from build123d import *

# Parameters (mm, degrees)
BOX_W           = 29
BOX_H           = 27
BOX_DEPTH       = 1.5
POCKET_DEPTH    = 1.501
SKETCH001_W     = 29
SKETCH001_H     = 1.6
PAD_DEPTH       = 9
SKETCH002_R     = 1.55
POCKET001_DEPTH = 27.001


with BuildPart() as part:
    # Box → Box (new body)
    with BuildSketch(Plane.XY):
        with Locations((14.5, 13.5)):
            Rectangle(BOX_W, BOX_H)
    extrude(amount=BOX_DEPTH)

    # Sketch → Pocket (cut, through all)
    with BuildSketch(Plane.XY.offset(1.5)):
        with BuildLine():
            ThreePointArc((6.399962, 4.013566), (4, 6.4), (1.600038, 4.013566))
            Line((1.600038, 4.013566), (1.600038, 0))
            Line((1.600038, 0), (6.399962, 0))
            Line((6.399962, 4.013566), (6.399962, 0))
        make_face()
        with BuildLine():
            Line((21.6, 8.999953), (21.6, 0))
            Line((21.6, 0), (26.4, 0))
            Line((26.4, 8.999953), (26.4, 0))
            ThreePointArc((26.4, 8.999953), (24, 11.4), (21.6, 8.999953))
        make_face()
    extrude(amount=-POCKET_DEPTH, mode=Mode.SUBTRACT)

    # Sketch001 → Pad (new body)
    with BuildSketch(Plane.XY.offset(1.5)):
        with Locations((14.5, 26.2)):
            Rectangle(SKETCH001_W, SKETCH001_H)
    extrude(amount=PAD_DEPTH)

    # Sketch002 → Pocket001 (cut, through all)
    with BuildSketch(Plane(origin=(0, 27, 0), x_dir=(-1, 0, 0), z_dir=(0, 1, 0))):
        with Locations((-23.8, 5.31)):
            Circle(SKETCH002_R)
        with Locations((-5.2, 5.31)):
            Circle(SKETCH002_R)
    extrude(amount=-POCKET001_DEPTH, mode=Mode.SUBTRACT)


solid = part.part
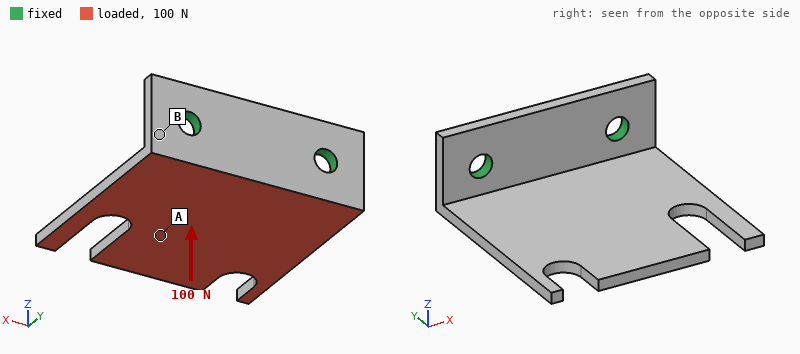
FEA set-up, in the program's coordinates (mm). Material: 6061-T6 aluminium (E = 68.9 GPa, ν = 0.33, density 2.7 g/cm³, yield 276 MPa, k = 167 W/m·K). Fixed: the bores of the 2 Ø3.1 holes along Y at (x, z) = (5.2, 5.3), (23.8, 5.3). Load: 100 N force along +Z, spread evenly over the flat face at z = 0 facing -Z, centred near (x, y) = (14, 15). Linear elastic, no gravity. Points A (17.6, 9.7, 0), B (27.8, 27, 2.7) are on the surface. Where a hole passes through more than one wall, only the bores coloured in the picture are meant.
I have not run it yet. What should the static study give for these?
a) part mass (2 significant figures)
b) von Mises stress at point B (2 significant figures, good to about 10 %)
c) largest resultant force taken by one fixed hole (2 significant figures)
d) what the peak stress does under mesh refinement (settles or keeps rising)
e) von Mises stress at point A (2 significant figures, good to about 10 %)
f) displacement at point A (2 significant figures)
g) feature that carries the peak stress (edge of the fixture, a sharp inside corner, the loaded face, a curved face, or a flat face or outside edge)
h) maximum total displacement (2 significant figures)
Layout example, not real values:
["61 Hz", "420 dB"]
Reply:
["3.9 g", "76 MPa", "52 N", "keeps rising", "17 MPa", "0.27 mm", "edge of the fixture", "0.48 mm"]
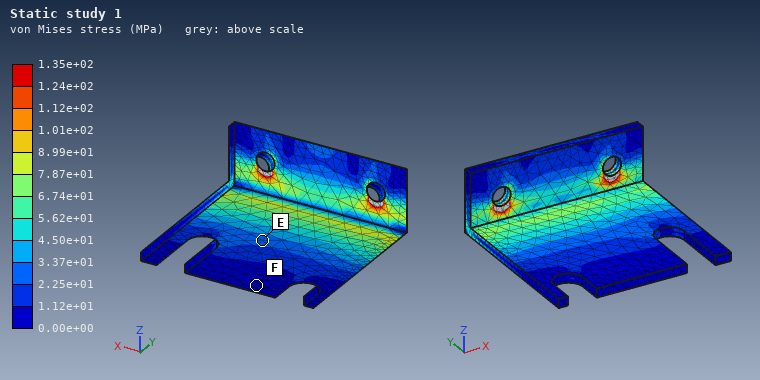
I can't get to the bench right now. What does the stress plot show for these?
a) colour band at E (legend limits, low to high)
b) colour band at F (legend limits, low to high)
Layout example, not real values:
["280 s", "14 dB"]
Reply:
["2.25e+01 to 3.37e+01 MPa", "0.00e+00 to 1.12e+01 MPa"]
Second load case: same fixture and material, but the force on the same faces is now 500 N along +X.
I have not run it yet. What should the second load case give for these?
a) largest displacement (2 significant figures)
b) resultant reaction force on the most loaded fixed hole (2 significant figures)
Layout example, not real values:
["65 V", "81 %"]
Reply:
["97 µm", "400 N"]
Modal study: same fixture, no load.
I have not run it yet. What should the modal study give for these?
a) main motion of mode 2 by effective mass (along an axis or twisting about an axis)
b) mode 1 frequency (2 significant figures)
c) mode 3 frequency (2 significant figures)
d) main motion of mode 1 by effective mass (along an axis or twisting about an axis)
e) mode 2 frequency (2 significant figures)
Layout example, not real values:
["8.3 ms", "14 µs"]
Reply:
["twisting about Y", "1700 Hz", "6700 Hz", "along Z", "3900 Hz"]
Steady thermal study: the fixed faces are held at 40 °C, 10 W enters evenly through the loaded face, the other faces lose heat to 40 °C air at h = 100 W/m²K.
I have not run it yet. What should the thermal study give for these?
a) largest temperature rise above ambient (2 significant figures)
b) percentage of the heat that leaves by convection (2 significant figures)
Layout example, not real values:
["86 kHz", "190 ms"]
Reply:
["20 K", "14 %"]
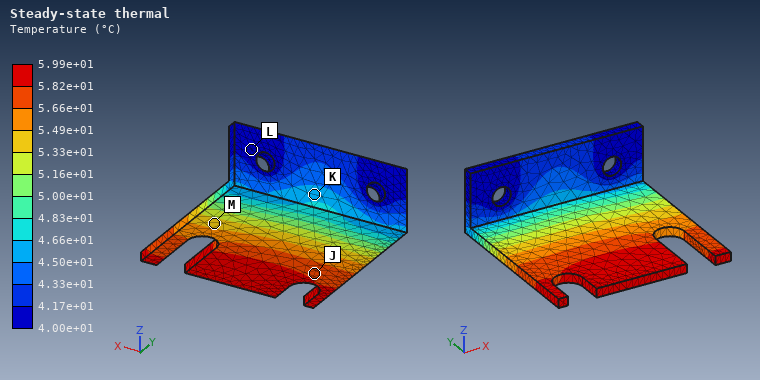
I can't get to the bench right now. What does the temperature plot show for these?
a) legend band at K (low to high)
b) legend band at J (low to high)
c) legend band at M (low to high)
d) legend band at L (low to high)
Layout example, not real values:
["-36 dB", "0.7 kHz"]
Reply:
["4.50e+01 to 4.66e+01 °C", "5.66e+01 to 5.82e+01 °C", "5.33e+01 to 5.49e+01 °C", "4.00e+01 to 4.17e+01 °C"]
